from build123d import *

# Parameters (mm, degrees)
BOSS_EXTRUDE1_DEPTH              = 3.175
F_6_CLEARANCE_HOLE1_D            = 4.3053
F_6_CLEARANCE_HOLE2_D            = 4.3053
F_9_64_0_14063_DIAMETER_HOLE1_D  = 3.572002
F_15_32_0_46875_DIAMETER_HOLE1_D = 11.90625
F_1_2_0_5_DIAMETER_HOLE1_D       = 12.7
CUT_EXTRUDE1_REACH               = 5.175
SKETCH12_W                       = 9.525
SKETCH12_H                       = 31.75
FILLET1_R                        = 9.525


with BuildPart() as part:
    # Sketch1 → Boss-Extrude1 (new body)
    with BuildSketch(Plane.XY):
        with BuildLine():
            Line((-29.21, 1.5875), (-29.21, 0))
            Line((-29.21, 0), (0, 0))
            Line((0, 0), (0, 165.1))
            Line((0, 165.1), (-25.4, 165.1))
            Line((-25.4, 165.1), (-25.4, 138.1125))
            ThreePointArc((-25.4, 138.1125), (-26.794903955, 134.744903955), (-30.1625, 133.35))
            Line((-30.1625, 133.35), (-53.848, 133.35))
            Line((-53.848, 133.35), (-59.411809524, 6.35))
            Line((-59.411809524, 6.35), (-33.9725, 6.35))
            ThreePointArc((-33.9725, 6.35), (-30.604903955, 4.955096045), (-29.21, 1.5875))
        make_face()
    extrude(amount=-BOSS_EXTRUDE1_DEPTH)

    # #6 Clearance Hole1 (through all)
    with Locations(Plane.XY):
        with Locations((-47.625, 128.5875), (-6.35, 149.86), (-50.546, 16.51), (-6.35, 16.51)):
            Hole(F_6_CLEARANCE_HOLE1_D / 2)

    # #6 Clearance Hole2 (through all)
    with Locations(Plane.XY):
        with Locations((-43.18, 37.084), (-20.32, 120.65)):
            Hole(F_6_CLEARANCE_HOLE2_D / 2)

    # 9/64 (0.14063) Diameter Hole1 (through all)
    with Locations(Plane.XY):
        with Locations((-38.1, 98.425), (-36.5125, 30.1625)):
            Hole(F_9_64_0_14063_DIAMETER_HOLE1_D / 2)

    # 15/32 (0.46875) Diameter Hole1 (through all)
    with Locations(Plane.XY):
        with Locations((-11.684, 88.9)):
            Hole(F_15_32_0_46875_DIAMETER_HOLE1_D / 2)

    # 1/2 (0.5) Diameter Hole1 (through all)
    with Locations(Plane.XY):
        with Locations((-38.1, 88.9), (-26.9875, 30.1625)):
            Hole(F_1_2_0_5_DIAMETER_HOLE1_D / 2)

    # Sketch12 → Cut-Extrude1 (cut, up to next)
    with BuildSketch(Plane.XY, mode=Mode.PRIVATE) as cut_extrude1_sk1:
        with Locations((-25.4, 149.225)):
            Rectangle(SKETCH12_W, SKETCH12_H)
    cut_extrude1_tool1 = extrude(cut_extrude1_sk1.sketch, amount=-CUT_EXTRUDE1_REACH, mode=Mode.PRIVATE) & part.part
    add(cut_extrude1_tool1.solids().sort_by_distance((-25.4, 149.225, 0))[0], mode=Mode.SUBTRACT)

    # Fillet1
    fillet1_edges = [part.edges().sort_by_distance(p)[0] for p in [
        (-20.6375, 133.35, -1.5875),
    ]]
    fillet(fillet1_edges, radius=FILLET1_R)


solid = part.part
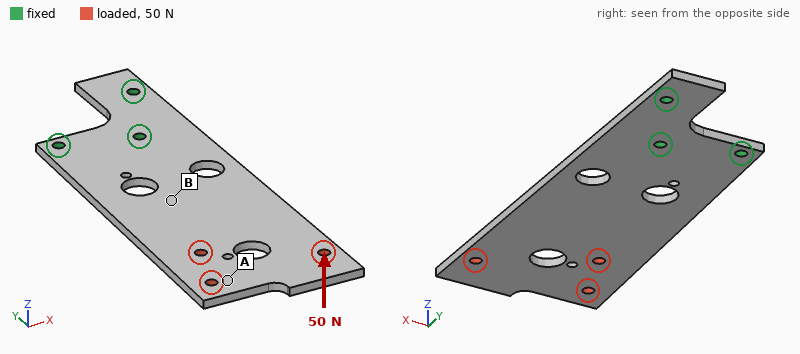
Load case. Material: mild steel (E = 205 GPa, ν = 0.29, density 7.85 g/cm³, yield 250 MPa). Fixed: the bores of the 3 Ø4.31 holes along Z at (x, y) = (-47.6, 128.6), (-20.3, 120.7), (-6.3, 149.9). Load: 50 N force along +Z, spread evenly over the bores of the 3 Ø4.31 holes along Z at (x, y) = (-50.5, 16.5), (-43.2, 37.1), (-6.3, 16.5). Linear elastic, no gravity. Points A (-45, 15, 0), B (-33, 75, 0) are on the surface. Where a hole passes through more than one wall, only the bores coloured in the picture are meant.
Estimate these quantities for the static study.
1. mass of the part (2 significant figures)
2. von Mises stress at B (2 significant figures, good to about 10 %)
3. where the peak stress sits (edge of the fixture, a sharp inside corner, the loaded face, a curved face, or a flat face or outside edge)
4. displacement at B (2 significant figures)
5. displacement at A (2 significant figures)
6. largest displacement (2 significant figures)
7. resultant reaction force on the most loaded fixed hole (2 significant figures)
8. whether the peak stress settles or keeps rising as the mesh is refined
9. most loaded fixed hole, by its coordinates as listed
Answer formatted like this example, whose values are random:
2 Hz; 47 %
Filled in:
190 g; 24 MPa; edge of the fixture; 0.18 mm; 0.69 mm; 0.82 mm; 110 N; keeps rising; (-20.3, 120.7)
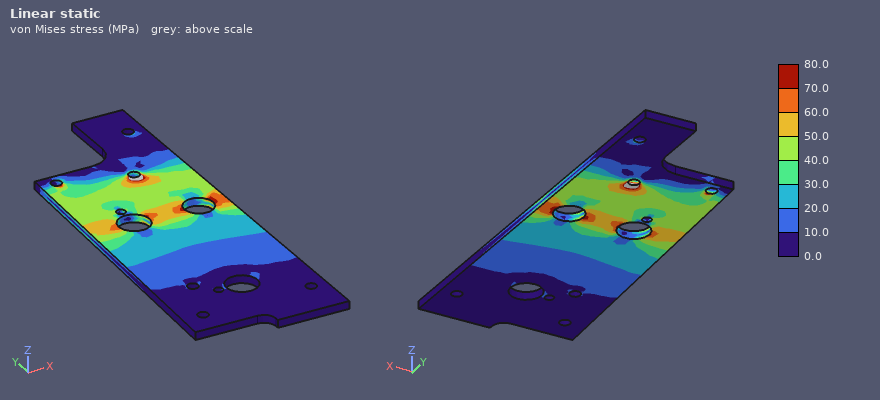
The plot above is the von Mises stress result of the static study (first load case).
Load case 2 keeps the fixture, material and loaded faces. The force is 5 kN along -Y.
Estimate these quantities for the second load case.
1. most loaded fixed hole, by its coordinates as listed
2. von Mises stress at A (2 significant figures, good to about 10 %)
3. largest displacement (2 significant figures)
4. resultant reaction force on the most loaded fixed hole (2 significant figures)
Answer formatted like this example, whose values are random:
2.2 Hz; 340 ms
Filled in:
(-47.6, 128.6); 18 MPa; 35 µm; 2.5 kN
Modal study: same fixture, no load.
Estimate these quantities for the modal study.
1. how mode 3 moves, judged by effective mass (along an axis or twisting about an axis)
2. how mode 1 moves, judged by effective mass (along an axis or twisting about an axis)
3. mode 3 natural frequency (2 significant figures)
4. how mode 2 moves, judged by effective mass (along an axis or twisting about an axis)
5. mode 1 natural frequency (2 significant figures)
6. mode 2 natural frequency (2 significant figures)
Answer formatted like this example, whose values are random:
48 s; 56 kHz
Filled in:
along Z; along Z; 1100 Hz; twisting about Y; 170 Hz; 730 Hz
